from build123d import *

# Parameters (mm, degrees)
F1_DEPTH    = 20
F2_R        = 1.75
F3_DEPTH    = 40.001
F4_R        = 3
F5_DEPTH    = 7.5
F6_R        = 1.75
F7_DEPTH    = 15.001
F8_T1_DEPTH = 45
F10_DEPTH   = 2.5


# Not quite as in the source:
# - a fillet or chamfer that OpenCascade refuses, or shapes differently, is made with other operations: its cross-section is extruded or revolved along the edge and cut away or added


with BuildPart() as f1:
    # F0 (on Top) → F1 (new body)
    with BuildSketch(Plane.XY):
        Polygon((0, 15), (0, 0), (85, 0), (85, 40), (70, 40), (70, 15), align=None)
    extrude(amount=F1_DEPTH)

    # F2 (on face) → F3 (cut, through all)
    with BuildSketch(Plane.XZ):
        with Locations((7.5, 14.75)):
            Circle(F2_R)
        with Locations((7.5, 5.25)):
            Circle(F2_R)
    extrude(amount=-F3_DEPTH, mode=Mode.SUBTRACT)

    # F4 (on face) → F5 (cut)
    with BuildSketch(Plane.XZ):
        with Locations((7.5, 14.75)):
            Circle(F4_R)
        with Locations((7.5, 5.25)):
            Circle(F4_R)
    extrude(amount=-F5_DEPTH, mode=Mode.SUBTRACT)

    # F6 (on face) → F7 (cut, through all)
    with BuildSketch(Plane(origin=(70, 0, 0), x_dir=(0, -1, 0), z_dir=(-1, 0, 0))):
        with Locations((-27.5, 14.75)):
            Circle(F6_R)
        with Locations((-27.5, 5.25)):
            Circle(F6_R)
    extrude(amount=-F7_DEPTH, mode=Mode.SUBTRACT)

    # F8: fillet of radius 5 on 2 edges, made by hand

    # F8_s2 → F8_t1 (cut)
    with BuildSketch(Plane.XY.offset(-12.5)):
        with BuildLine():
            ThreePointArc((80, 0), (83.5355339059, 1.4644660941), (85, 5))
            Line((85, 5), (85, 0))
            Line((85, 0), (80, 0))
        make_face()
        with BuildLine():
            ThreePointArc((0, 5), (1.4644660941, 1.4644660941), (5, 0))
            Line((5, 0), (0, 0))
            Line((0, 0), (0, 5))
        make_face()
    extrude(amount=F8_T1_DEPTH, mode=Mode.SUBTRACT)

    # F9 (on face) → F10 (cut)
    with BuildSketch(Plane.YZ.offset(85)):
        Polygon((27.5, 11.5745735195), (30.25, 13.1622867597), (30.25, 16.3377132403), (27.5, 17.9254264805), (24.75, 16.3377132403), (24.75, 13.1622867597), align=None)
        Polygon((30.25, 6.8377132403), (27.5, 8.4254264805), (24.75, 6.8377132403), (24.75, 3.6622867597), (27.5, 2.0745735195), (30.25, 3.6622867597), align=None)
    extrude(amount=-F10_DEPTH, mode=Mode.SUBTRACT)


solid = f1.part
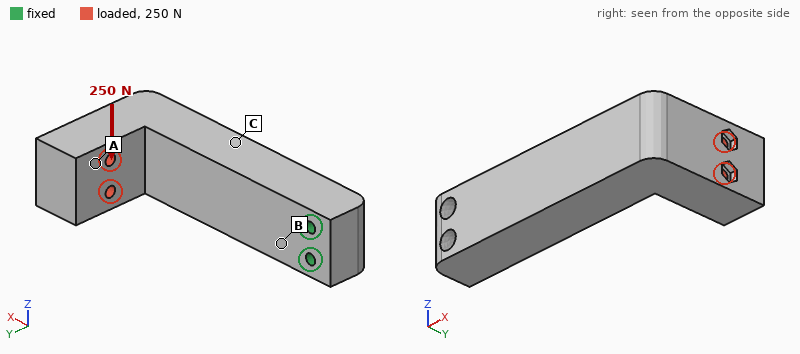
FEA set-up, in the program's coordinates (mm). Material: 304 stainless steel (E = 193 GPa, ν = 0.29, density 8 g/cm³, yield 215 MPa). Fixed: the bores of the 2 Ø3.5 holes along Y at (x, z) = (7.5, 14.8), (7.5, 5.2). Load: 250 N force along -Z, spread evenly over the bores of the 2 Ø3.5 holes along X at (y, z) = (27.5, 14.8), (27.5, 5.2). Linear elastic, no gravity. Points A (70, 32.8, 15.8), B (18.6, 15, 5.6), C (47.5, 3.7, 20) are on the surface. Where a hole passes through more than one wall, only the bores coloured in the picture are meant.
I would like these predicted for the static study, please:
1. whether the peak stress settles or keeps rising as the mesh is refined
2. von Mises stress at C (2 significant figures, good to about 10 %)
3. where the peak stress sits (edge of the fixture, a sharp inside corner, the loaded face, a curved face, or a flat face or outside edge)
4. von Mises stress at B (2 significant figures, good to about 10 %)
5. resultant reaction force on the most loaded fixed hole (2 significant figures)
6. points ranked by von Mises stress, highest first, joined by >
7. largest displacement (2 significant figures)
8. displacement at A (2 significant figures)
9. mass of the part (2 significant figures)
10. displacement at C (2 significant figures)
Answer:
keeps rising
9.3 MPa
edge of the fixture
15 MPa
1.5 kN
B > C > A
37 µm
28 µm
250 g
9.1 µm
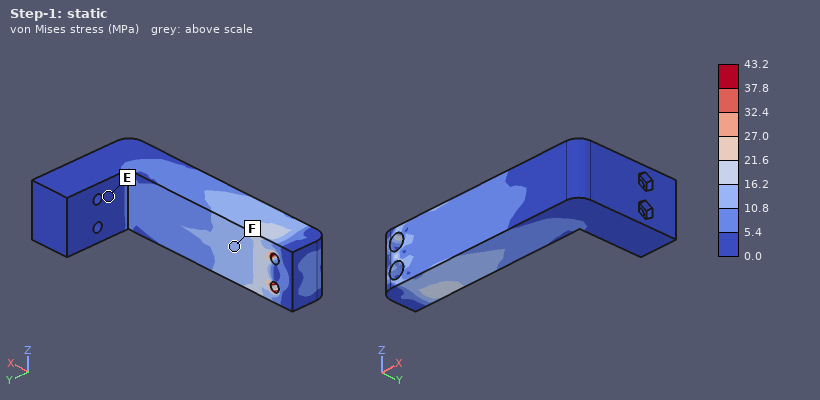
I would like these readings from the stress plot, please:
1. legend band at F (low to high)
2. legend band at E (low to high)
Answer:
10.8 to 16.2 MPa
0.0 to 5.4 MPa
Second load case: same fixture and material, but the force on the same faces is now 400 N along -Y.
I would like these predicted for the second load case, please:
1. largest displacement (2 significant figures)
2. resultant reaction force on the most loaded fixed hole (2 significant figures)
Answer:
90 µm
240 N
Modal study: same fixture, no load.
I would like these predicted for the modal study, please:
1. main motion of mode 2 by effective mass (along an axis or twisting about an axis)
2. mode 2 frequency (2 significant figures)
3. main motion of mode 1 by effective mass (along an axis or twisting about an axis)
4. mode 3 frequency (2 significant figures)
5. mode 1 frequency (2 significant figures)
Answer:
along Z
1500 Hz
along Y
4000 Hz
1000 Hz
